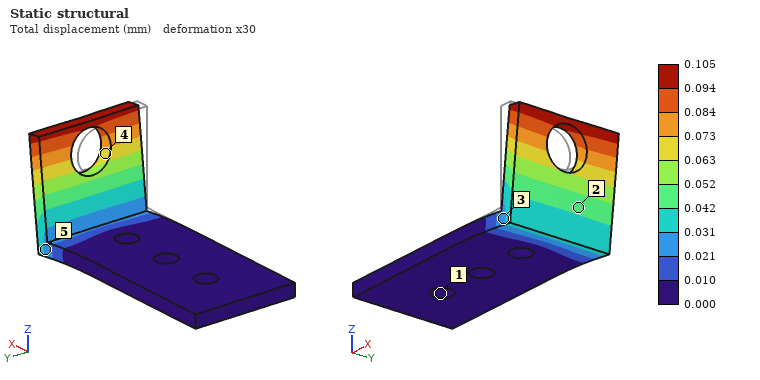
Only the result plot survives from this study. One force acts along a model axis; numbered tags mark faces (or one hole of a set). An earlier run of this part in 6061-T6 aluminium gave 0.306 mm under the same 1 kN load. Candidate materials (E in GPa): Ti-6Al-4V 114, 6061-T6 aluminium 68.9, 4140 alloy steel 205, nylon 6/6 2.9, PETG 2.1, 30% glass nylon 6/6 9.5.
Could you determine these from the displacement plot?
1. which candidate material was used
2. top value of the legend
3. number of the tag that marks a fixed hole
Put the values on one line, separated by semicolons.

4140 alloy steel; 0.105 mm; 1
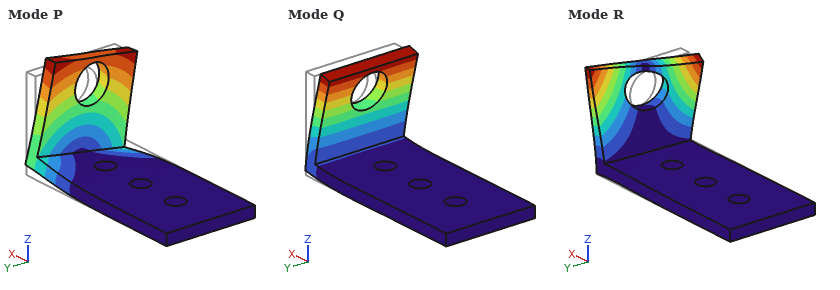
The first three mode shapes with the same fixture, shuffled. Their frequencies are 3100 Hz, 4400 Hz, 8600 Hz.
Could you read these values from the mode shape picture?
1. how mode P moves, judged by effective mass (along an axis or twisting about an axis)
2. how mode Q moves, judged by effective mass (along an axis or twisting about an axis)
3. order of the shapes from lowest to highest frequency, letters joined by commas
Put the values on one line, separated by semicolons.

along Y; along X; Q, P, R
